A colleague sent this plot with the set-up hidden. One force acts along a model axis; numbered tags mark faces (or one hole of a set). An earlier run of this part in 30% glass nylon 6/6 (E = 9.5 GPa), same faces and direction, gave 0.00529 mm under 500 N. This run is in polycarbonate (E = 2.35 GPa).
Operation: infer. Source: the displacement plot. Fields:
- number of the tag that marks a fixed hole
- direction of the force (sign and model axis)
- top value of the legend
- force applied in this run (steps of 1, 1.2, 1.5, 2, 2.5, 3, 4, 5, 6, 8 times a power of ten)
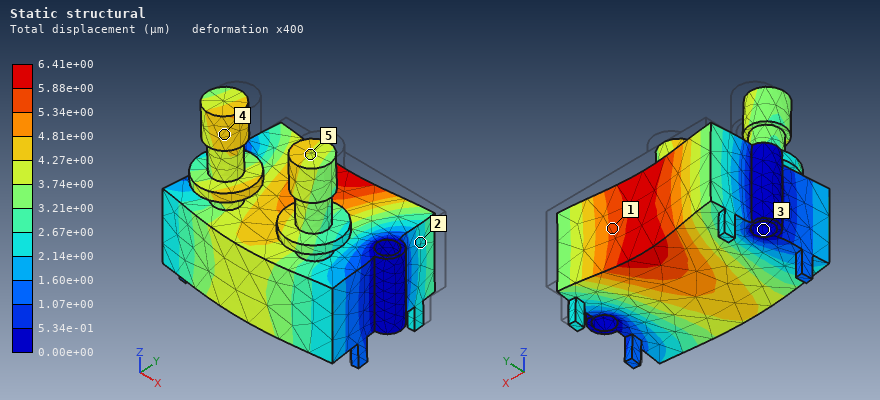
3
-Y
6.41e+00 µm
150 N
